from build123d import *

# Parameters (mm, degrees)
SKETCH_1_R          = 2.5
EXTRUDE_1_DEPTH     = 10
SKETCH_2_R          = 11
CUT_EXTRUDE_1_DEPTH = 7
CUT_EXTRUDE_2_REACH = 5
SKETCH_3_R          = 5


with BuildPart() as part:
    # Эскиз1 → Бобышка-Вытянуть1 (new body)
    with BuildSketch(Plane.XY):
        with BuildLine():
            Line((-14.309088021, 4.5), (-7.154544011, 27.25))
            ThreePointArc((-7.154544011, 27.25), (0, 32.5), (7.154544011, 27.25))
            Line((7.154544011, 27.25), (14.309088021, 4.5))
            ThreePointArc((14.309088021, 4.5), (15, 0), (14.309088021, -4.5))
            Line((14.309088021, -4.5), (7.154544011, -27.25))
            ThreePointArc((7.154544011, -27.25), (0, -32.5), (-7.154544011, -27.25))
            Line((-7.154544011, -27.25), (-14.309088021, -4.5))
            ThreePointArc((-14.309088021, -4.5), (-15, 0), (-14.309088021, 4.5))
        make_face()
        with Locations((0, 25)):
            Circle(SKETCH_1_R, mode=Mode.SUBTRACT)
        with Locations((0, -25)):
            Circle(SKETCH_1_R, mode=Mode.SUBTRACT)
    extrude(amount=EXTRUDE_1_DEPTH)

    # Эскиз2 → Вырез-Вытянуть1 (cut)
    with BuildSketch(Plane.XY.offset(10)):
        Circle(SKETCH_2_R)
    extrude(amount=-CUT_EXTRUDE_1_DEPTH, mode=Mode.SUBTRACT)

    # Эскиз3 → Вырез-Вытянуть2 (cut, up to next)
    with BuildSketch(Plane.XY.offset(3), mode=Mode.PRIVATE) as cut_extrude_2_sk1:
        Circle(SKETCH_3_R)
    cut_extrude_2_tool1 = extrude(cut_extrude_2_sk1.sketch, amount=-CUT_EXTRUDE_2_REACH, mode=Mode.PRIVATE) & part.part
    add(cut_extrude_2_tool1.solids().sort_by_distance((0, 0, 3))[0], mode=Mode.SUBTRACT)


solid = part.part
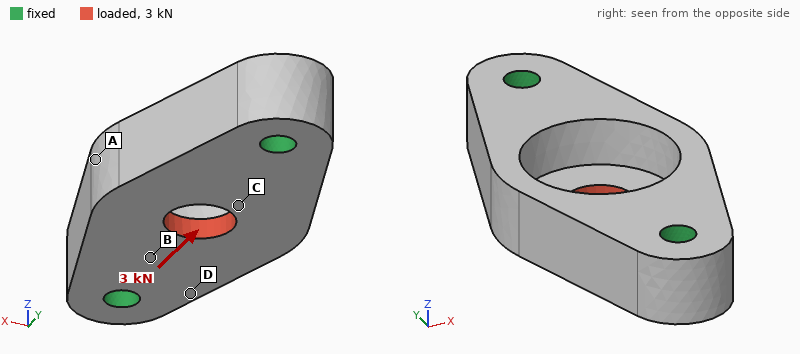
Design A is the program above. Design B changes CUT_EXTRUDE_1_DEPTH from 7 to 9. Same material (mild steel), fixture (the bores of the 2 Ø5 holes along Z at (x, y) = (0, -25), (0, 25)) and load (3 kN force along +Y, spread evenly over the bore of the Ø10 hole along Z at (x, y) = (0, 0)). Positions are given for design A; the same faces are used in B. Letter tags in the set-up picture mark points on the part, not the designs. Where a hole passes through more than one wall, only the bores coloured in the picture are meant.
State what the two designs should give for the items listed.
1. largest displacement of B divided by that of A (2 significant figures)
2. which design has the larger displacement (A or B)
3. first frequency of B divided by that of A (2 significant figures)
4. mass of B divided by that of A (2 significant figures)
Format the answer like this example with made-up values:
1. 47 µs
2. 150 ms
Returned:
1. 2.2
2. B
3. 1.0
4. 0.94
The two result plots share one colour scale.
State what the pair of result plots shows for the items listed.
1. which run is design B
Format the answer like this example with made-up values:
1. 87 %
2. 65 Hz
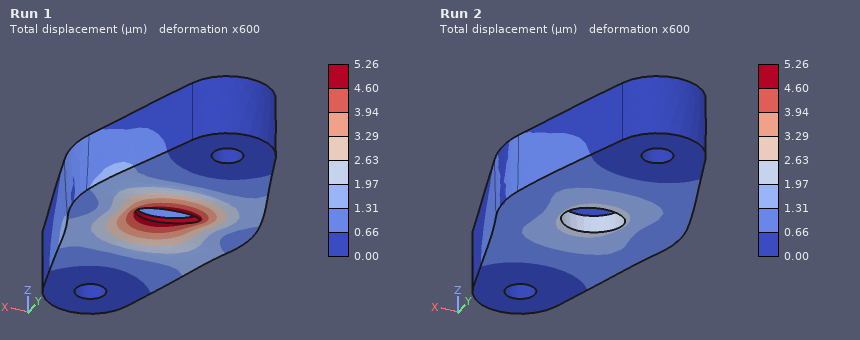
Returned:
1. Run 1
